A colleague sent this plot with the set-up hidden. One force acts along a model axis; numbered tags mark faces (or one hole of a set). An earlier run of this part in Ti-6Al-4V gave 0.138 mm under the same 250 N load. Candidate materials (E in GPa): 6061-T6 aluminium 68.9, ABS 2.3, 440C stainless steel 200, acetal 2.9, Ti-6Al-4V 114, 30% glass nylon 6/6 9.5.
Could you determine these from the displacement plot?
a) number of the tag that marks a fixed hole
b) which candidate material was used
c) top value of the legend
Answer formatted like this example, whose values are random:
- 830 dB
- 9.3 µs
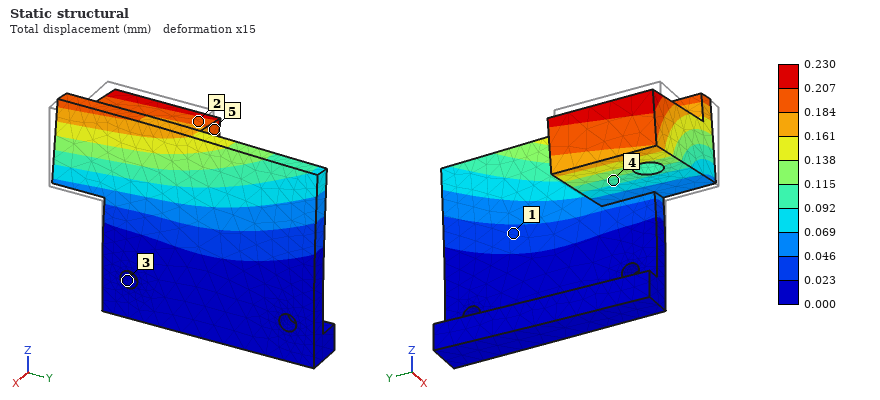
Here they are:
- 3
- 6061-T6 aluminium
- 0.230 mm
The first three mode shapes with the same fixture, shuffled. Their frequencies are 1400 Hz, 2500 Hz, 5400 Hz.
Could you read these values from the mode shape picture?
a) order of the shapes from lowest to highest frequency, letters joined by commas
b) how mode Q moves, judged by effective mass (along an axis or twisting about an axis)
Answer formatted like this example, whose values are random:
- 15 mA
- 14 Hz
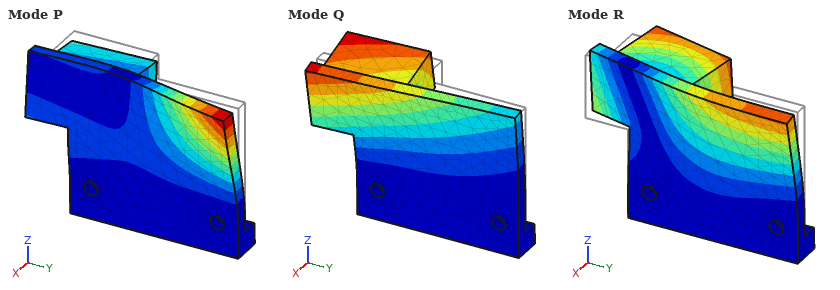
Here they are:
- Q, R, P
- along X
